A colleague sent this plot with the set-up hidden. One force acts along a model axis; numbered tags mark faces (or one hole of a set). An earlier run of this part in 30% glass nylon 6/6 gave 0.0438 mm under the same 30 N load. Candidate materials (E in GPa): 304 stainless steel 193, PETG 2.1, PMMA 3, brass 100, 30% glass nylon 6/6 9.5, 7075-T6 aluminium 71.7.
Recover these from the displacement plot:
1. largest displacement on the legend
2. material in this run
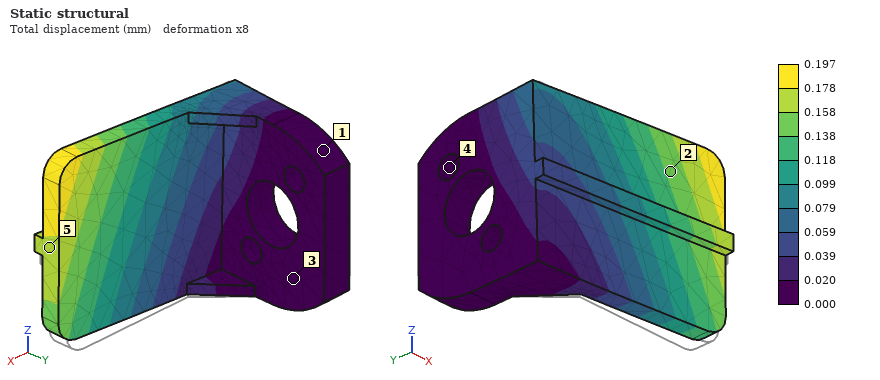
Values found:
0.197 mm
PETG
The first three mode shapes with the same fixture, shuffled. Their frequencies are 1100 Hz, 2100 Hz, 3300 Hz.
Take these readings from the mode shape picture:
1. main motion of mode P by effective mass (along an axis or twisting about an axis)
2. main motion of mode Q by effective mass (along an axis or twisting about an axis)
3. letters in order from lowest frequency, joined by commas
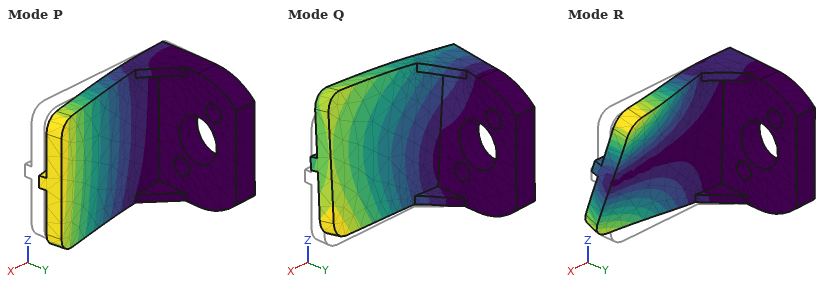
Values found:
along Y
along Z
P, Q, R
